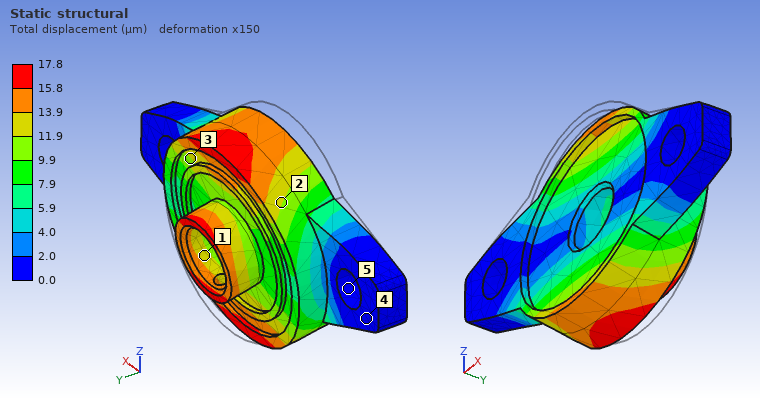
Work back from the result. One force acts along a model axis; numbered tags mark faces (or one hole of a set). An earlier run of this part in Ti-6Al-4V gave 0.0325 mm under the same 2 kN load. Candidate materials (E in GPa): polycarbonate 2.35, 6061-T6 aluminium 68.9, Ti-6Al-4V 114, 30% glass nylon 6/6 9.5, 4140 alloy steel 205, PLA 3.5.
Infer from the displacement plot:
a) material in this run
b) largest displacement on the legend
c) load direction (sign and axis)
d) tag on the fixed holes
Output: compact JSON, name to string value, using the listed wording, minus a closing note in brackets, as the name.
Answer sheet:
{"material in this run": "4140 alloy steel", "largest displacement on the legend": "17.8 µm", "load direction": "-Z", "tag on the fixed holes": "5"}
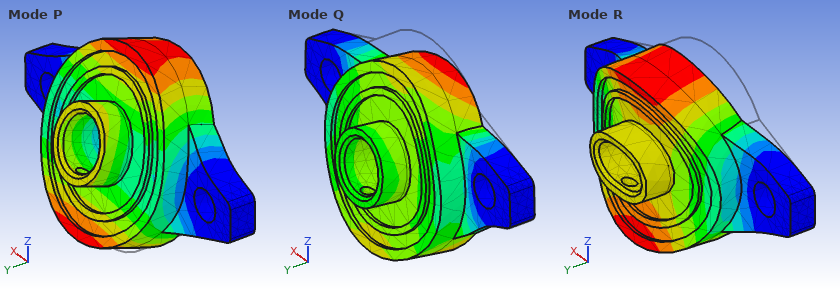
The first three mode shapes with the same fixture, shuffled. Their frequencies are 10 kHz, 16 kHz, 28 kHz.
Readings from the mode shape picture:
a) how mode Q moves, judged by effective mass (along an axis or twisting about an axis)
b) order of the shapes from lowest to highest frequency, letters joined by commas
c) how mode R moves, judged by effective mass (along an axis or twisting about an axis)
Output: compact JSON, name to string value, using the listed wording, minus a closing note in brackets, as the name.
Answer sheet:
{"how mode Q moves, judged by effective mass": "along Z", "order of the shapes from lowest to highest frequency, letters joined by commas": "P, R, Q", "how mode R moves, judged by effective mass": "along Y"}
